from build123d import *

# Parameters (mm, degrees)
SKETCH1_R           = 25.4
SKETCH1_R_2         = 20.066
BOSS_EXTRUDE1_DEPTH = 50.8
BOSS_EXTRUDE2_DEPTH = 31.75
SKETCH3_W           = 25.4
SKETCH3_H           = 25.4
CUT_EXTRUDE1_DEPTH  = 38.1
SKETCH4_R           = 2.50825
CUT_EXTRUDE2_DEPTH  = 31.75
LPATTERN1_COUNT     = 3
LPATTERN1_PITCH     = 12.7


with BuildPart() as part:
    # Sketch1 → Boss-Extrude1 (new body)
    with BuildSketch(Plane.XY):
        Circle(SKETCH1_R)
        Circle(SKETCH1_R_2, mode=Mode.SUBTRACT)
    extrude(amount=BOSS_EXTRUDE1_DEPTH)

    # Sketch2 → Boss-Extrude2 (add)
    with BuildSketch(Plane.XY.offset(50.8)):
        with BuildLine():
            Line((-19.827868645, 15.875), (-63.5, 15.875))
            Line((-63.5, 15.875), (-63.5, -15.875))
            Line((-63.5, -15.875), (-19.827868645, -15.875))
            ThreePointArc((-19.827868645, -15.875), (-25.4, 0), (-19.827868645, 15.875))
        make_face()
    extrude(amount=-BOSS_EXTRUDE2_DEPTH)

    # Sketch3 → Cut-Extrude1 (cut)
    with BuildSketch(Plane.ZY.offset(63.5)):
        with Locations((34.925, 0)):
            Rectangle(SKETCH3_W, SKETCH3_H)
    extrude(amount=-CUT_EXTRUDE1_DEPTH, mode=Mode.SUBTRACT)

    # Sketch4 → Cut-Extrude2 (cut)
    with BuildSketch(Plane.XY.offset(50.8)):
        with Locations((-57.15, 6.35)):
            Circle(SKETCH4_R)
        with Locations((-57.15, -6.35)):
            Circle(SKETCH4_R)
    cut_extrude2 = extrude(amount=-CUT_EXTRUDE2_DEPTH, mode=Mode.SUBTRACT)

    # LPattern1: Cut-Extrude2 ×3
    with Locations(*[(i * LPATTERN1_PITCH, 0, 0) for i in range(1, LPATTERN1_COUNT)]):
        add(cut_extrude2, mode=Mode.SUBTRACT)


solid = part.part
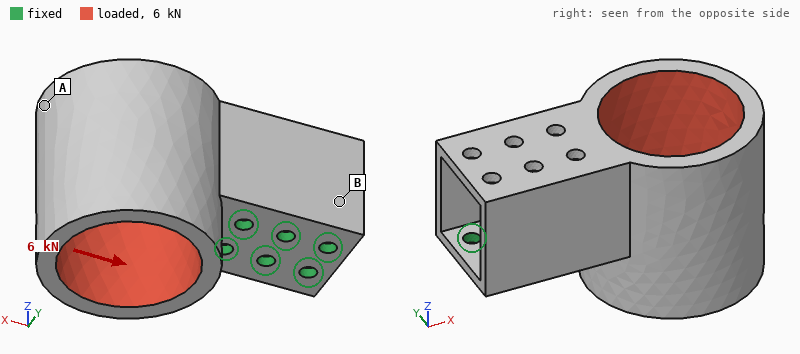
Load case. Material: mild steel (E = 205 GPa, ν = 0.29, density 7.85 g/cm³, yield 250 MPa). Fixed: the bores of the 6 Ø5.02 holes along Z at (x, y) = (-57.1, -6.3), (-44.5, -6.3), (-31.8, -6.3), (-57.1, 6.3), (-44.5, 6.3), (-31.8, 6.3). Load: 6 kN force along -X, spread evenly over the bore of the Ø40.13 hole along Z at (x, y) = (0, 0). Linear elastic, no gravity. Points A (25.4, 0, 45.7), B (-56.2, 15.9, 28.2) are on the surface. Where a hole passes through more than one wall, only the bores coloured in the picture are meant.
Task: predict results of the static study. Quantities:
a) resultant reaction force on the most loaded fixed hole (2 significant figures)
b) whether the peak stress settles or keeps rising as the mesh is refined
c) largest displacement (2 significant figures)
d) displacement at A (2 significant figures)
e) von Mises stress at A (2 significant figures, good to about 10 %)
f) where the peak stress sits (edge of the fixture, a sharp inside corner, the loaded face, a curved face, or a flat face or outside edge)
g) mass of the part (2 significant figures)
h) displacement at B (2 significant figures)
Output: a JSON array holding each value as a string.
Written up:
["2.0 kN", "keeps rising", "23 µm", "22 µm", "25 MPa", "edge of the fixture", "420 g", "5.1 µm"]
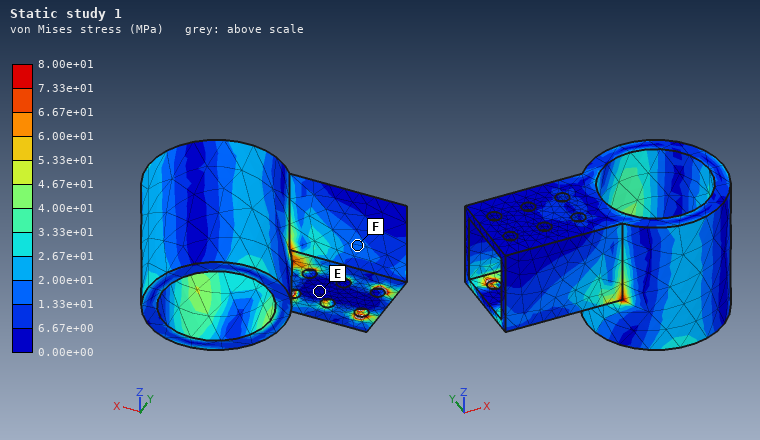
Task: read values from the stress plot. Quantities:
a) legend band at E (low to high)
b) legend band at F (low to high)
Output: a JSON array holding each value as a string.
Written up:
["0.00e+00 to 6.67e+00 MPa", "1.33e+01 to 2.00e+01 MPa"]
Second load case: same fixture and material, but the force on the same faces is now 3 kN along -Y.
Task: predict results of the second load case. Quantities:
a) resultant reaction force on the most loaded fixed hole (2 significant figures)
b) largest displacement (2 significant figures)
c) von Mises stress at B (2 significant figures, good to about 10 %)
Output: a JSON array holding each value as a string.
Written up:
["3.2 kN", "84 µm", "19 MPa"]
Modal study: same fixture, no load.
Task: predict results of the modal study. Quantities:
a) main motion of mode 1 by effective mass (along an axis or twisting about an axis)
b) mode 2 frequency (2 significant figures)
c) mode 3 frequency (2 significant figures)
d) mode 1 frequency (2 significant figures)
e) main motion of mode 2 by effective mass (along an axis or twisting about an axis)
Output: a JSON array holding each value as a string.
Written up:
["along Z", "1900 Hz", "2200 Hz", "1800 Hz", "along Y"]
